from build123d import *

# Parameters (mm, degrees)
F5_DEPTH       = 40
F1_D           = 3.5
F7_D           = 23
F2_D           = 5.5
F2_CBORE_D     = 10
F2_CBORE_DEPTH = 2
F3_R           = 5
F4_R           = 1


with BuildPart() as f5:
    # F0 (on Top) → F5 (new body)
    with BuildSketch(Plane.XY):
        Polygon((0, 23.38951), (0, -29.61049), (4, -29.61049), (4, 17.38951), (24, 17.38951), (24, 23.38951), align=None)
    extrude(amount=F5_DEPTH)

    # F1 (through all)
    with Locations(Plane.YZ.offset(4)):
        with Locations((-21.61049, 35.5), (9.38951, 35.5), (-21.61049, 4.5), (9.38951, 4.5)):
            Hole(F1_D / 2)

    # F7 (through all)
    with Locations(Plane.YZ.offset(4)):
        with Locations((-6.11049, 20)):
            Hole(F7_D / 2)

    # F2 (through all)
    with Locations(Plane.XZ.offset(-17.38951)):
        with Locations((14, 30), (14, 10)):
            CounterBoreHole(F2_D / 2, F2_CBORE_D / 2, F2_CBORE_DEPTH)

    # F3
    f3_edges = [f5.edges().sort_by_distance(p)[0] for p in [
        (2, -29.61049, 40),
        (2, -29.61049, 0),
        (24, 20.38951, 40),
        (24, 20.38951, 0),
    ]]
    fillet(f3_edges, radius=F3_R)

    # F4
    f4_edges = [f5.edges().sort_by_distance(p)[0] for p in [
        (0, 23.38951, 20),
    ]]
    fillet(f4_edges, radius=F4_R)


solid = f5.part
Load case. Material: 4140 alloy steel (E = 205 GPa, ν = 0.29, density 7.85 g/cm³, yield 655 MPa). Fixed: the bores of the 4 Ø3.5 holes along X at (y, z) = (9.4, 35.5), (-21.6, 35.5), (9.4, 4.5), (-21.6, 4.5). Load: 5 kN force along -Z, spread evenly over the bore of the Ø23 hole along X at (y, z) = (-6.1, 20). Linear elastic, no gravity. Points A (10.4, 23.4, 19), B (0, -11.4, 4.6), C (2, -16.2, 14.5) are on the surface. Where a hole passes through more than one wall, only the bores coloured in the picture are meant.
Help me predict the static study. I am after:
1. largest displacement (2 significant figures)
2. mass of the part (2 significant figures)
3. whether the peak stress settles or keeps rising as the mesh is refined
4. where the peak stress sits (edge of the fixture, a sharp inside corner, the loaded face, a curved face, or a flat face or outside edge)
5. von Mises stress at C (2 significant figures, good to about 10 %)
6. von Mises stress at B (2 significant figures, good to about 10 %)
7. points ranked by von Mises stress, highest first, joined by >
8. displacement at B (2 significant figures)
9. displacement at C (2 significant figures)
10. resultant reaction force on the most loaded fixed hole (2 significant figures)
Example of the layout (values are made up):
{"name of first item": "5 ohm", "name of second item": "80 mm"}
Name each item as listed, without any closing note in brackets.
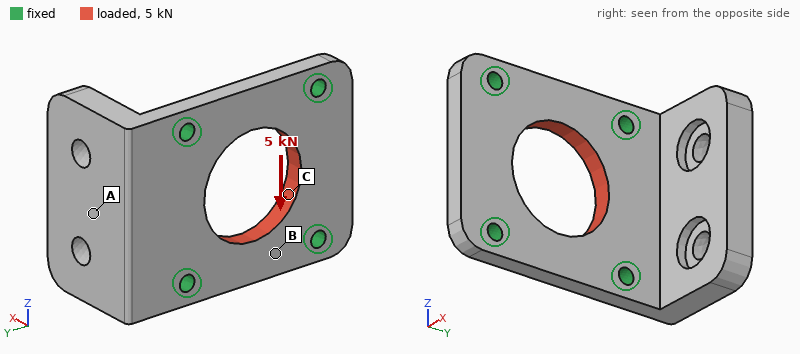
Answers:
{"largest displacement": "4.1 µm", "mass of the part": "85 g", "whether the peak stress settles or keeps rising as the mesh is refined": "keeps rising", "where the peak stress sits": "edge of the fixture", "von Mises stress at C": "40 MPa", "von Mises stress at B": "24 MPa", "points ranked by von Mises stress, highest first, joined by >": "C > B > A", "displacement at B": "3.1 µm", "displacement at C": "1.9 µm", "resultant reaction force on the most loaded fixed hole": "1.3 kN"}
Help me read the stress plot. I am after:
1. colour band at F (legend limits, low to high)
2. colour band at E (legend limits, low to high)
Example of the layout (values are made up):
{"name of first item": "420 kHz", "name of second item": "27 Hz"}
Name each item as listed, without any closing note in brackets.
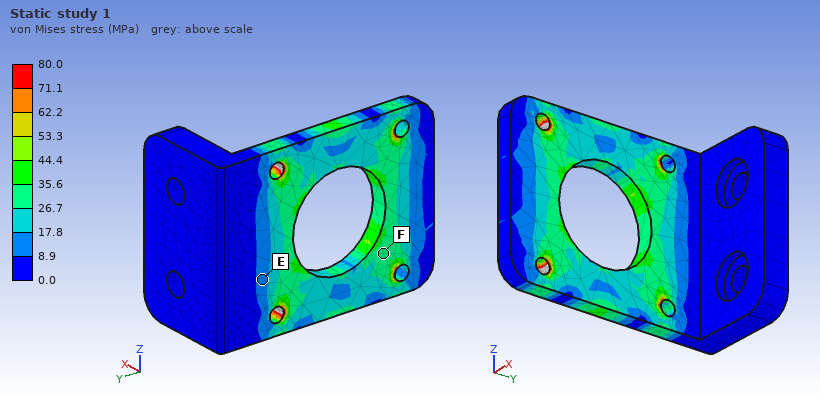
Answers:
{"colour band at F": "26.7 to 35.6 MPa", "colour band at E": "8.9 to 17.8 MPa"}
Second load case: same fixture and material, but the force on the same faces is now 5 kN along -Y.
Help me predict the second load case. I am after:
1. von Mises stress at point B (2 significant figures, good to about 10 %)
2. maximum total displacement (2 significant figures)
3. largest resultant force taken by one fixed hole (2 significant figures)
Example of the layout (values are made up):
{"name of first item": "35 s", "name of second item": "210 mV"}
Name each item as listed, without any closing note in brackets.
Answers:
{"von Mises stress at point B": "18 MPa", "maximum total displacement": "3.5 µm", "largest resultant force taken by one fixed hole": "1.3 kN"}
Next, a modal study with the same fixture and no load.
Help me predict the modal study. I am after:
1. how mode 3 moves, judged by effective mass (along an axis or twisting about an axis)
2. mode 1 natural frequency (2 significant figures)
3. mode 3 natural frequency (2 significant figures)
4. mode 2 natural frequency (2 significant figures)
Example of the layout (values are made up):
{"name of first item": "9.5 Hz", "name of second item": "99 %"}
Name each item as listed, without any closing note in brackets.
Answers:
{"how mode 3 moves, judged by effective mass": "along X", "mode 1 natural frequency": "3500 Hz", "mode 3 natural frequency": "12 kHz", "mode 2 natural frequency": "8100 Hz"}
